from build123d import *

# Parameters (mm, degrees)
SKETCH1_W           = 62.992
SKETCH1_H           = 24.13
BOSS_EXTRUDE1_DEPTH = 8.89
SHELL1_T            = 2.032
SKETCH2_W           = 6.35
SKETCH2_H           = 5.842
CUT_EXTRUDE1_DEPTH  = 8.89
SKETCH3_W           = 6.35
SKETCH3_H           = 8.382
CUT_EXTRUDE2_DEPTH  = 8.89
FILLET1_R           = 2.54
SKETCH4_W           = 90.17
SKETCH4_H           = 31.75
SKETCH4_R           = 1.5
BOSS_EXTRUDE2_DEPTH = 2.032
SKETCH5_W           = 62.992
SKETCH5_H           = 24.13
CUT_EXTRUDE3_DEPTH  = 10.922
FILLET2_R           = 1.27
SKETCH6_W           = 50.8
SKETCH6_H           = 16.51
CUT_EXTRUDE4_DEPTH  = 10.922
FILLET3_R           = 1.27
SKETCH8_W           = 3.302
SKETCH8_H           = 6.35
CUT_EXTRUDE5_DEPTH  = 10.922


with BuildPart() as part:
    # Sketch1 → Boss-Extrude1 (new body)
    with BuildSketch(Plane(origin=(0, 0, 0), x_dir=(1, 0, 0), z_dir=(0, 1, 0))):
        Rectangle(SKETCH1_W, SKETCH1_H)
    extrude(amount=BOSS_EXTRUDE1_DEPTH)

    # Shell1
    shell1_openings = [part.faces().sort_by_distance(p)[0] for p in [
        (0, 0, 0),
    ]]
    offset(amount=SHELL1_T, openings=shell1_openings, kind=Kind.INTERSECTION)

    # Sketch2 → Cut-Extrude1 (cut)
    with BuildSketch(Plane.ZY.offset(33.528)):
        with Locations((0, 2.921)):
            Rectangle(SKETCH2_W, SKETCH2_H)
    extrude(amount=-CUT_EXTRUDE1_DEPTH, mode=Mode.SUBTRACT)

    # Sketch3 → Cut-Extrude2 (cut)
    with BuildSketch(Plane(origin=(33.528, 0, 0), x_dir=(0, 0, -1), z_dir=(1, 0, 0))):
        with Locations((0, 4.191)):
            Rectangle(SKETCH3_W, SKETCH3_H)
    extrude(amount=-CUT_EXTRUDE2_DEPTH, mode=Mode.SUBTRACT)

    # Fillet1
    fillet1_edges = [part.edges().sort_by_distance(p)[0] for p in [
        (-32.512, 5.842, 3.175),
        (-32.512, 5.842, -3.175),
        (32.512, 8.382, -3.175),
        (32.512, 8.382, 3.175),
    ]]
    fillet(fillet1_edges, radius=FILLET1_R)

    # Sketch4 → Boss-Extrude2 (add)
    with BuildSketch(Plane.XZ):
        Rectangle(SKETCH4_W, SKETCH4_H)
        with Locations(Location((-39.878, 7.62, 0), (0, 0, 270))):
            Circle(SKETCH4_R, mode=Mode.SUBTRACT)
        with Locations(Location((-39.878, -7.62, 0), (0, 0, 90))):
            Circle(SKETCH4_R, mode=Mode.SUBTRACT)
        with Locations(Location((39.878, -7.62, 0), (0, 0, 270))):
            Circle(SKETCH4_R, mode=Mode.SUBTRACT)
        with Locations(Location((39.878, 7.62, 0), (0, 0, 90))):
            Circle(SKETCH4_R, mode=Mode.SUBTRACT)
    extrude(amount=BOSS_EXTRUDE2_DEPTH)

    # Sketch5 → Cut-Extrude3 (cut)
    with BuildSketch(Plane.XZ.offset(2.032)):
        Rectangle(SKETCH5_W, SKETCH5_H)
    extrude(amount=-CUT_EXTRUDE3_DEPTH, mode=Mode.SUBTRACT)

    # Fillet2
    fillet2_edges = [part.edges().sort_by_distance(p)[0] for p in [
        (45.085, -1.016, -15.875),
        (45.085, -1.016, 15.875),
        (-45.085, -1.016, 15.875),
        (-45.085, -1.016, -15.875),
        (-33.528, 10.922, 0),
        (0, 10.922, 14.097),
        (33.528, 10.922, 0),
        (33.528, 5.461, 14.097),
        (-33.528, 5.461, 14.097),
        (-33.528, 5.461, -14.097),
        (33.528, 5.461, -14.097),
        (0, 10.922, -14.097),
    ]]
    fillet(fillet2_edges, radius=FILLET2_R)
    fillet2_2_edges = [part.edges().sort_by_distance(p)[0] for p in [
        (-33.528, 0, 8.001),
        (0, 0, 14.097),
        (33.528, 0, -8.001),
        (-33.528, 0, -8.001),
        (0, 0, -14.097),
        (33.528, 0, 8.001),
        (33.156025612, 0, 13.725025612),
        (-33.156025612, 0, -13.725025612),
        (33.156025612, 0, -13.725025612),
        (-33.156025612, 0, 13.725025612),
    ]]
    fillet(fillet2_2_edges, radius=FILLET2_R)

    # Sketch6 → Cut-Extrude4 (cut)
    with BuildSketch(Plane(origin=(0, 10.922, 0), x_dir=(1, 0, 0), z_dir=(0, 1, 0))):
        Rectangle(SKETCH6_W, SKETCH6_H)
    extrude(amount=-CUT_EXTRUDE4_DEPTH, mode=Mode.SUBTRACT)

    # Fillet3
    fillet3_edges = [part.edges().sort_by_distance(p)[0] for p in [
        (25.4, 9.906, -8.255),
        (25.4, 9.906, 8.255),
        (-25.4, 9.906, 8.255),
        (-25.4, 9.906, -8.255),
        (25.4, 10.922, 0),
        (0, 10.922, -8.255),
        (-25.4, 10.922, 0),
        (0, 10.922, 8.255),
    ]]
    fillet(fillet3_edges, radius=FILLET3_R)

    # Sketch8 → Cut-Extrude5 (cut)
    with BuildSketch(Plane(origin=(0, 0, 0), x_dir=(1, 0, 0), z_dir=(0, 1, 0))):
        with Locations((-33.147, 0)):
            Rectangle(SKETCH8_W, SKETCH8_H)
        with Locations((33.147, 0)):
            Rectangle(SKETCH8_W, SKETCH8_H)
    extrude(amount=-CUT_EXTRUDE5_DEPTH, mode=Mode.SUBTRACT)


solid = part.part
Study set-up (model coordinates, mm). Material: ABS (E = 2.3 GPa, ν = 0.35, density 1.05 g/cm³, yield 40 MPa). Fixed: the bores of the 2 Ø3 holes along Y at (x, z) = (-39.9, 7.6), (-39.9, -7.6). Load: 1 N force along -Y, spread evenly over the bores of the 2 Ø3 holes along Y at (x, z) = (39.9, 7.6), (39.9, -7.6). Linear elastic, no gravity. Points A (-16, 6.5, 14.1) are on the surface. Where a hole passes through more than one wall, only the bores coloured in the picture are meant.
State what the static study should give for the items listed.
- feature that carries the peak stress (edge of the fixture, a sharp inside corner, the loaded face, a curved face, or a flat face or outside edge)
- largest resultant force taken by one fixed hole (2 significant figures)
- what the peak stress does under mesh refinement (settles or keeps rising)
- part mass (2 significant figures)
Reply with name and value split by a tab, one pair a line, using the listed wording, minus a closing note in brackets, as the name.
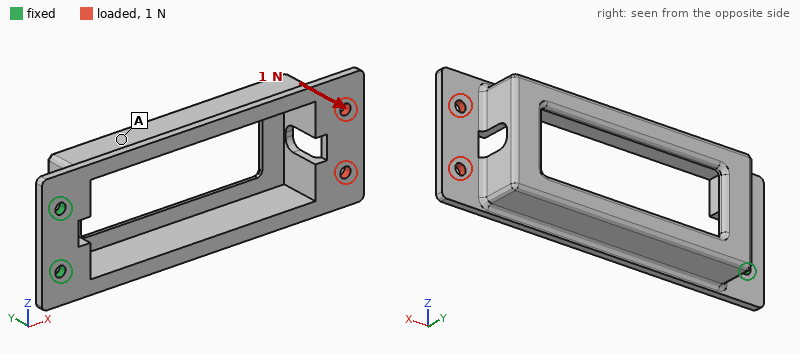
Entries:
feature that carries the peak stress	edge of the fixture
largest resultant force taken by one fixed hole	1.4 N
what the peak stress does under mesh refinement	keeps rising
part mass	8.2 g
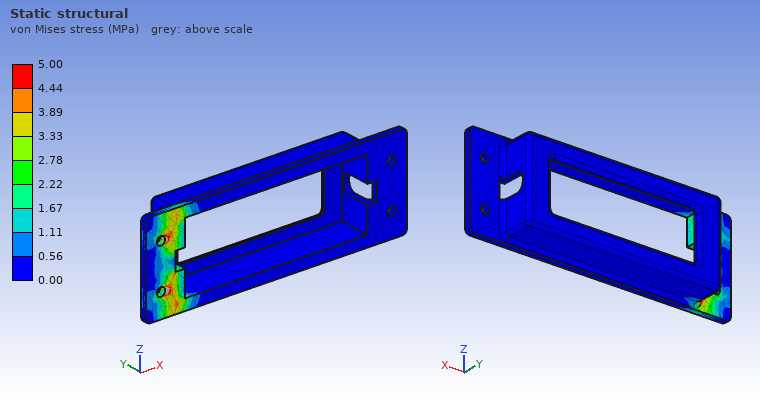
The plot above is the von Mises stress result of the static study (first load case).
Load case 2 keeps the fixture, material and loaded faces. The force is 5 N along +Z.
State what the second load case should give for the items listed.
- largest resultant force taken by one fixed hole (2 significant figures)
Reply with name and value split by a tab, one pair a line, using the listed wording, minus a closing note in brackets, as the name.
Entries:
largest resultant force taken by one fixed hole	20 N
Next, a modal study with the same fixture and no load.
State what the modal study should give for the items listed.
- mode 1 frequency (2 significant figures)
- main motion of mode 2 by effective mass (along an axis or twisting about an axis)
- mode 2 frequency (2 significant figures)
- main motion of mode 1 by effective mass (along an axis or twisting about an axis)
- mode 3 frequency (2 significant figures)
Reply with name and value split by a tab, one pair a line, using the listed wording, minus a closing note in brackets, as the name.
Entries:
mode 1 frequency	94 Hz
main motion of mode 2 by effective mass	along Z
mode 2 frequency	210 Hz
main motion of mode 1 by effective mass	along Y
mode 3 frequency	550 Hz
